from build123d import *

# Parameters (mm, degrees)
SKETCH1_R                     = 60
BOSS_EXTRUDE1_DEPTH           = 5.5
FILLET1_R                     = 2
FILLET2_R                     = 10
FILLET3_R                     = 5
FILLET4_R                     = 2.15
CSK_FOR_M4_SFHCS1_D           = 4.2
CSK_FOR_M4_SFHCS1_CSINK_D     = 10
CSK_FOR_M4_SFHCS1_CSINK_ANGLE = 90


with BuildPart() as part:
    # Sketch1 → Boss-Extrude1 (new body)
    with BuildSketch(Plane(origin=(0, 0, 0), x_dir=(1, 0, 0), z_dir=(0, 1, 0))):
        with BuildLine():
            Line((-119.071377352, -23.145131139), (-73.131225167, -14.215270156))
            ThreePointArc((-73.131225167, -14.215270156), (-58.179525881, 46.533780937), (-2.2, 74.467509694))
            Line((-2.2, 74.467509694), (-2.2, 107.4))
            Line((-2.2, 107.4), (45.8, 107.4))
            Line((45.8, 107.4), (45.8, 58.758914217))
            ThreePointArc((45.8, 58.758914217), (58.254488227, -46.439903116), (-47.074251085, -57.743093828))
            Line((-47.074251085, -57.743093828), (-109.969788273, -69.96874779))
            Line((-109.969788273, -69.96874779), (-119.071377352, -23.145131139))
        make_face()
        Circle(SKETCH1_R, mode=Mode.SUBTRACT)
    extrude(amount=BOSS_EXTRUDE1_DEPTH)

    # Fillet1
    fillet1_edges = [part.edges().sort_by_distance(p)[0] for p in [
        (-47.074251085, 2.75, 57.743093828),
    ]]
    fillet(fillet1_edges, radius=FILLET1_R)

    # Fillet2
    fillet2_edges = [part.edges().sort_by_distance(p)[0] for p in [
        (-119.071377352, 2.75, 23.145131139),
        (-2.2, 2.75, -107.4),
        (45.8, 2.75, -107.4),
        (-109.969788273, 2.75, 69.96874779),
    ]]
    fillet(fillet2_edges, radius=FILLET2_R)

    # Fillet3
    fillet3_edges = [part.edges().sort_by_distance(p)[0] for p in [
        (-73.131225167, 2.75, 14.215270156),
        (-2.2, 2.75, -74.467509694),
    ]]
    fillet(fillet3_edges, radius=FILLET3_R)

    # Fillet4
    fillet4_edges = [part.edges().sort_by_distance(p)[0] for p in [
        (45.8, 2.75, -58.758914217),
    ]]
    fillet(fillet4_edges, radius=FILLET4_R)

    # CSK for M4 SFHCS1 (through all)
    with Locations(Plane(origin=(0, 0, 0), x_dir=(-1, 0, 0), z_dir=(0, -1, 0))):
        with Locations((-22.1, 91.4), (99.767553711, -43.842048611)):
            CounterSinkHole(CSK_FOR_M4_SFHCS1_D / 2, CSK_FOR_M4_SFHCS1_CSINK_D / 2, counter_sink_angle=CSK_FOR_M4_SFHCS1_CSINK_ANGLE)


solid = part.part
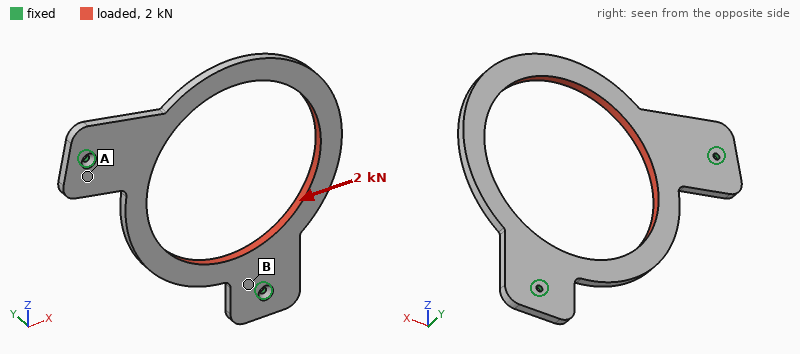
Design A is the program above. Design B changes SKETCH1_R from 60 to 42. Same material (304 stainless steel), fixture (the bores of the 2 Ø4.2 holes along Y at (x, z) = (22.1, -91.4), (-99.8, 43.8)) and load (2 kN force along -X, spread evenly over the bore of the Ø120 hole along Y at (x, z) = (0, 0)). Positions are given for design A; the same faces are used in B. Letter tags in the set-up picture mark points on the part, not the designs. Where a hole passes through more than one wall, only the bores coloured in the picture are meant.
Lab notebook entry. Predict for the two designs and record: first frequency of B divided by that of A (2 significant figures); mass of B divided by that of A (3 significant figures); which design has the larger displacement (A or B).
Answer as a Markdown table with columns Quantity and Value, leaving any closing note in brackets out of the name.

| Quantity | Value |
|---|---|
| first frequency of B divided by that of A | 0.88 |
| mass of B divided by that of A | 1.56 |
| which design has the larger displacement | A |
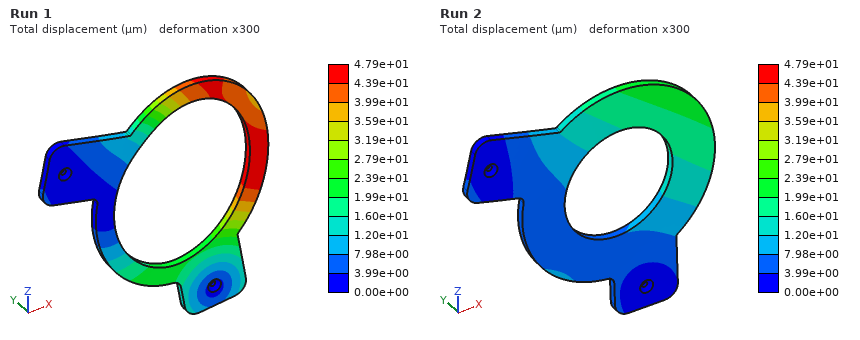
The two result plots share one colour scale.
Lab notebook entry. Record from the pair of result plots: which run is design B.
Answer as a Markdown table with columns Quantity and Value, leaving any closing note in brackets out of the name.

| Quantity | Value |
|---|---|
| which run is design B | Run 2 |
